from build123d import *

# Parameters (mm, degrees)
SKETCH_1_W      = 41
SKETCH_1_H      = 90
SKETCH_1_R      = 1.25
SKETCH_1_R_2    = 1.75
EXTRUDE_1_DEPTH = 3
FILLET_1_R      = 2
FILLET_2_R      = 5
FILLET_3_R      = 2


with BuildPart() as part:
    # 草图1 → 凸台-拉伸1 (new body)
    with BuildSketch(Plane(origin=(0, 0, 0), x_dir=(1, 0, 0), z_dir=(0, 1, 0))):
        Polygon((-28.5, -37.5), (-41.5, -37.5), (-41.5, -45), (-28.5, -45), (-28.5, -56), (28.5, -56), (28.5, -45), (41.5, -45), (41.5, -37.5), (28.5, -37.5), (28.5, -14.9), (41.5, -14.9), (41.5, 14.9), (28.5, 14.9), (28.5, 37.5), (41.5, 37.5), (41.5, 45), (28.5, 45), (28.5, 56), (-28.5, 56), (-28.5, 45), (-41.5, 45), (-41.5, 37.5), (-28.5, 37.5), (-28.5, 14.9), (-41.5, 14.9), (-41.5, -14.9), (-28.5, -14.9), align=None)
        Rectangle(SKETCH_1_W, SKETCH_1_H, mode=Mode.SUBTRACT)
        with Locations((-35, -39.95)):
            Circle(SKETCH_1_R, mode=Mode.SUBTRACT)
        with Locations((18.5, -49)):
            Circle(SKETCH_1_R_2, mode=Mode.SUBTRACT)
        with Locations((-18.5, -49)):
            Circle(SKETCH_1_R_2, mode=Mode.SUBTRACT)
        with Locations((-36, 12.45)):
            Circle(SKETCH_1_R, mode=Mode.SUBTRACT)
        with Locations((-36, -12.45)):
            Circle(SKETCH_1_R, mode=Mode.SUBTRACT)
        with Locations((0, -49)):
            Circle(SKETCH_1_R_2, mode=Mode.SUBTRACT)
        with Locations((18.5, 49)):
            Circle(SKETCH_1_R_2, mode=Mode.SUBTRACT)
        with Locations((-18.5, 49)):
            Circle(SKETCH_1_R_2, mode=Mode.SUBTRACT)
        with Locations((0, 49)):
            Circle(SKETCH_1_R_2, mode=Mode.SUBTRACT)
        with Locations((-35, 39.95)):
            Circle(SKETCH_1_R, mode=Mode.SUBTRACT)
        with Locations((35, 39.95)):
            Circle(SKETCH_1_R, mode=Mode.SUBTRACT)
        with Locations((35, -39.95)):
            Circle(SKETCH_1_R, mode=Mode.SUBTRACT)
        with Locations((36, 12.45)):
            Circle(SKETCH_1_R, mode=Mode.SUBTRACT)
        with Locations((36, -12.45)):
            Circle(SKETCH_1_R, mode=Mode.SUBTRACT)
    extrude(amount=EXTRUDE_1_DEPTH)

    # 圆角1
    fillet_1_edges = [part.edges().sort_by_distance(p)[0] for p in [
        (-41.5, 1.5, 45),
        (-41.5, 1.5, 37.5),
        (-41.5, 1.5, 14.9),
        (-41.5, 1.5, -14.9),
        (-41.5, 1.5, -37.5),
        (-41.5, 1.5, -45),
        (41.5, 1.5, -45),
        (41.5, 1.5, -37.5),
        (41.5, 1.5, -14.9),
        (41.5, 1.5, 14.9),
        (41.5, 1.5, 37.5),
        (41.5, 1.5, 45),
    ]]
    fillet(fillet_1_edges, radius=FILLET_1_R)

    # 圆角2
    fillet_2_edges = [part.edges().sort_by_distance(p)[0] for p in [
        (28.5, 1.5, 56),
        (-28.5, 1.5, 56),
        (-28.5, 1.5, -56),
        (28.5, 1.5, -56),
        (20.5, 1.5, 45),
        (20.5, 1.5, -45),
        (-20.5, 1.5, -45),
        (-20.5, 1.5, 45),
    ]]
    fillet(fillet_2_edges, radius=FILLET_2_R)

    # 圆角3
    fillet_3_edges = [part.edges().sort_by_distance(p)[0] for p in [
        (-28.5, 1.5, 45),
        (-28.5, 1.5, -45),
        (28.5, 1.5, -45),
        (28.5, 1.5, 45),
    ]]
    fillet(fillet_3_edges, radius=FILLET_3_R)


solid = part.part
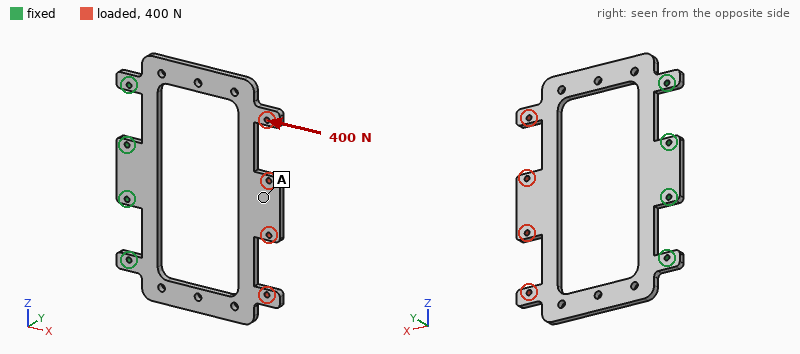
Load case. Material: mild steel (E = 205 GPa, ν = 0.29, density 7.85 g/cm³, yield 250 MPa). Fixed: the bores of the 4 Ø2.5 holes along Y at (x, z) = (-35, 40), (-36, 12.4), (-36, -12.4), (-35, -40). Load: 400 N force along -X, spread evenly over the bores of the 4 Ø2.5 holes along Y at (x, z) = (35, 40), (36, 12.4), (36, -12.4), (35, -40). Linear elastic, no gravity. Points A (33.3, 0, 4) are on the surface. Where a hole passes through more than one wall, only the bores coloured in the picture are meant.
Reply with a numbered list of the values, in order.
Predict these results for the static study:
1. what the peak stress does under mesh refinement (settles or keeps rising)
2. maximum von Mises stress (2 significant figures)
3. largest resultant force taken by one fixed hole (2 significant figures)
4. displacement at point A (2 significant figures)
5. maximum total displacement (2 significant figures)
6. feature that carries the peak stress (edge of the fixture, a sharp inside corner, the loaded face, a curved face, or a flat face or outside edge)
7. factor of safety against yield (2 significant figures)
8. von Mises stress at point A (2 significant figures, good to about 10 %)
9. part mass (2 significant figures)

1. settles
2. 75 MPa
3. 250 N
4. 36 µm
5. 36 µm
6. a curved face
7. 3.3
8. 7.9 MPa
9. 88 g
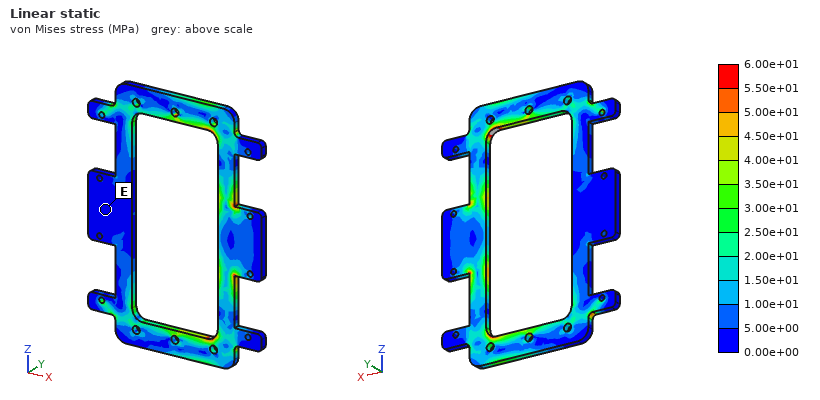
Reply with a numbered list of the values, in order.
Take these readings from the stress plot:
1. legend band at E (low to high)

1. 0.00e+00 to 5.00e+00 MPa
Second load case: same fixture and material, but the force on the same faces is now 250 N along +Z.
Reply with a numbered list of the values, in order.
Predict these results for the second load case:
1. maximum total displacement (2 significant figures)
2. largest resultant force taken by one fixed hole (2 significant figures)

1. 96 µm
2. 340 N
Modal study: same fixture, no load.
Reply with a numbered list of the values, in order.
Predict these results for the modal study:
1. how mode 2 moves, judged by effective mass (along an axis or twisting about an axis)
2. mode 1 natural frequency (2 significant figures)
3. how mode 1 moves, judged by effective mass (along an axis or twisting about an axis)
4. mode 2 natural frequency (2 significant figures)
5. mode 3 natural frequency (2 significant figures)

1. twisting about X
2. 250 Hz
3. along Y
4. 570 Hz
5. 1200 Hz
